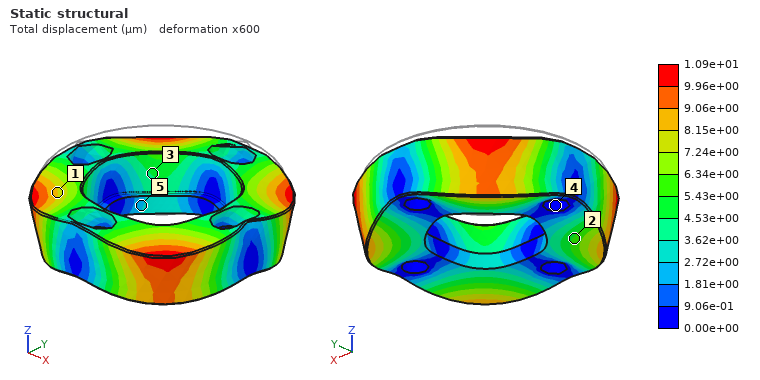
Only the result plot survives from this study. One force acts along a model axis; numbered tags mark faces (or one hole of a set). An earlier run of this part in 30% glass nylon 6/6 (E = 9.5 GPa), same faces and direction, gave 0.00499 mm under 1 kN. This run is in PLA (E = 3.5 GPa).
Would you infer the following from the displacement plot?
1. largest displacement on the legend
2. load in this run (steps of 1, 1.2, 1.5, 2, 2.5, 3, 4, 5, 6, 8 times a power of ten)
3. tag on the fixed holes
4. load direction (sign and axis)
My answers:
1.09e+01 µm
800 N
4
-Z
